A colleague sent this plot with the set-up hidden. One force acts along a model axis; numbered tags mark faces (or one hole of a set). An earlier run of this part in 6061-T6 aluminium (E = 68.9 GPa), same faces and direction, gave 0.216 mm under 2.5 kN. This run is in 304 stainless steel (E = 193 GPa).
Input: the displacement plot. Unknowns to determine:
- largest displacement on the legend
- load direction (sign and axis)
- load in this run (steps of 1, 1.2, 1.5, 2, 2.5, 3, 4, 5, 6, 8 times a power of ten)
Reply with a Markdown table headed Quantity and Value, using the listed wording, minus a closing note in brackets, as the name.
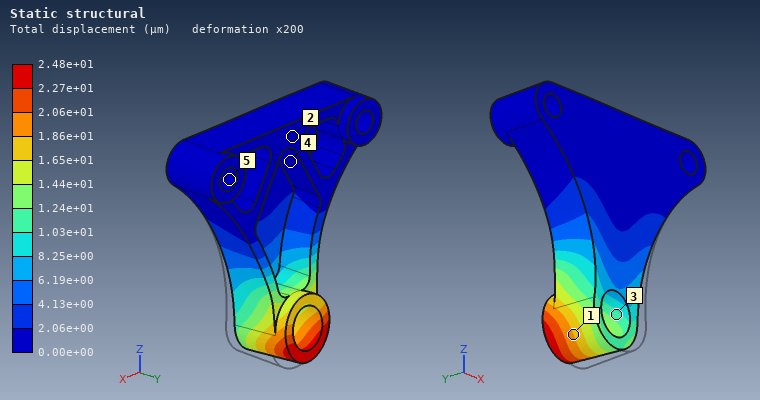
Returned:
| Quantity | Value |
|---|---|
| largest displacement on the legend | 2.48e+01 µm |
| load direction | -X |
| load in this run | 800 N |
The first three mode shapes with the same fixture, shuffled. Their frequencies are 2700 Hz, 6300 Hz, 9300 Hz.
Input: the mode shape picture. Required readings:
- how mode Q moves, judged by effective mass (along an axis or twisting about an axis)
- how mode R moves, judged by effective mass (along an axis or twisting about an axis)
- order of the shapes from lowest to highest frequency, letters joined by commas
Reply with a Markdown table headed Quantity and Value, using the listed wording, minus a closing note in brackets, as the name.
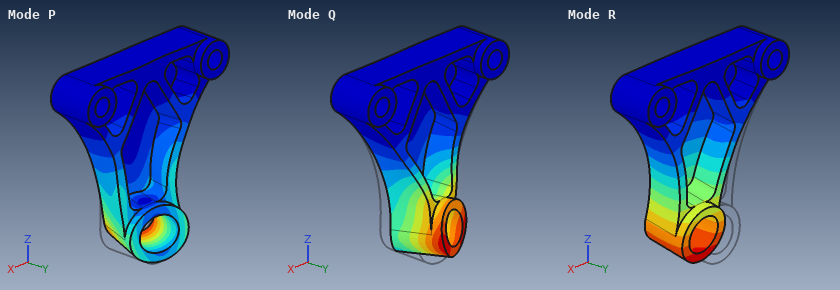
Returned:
| Quantity | Value |
|---|---|
| how mode Q moves, judged by effective mass | along X |
| how mode R moves, judged by effective mass | along Y |
| order of the shapes from lowest to highest frequency, letters joined by commas | R, Q, P |
